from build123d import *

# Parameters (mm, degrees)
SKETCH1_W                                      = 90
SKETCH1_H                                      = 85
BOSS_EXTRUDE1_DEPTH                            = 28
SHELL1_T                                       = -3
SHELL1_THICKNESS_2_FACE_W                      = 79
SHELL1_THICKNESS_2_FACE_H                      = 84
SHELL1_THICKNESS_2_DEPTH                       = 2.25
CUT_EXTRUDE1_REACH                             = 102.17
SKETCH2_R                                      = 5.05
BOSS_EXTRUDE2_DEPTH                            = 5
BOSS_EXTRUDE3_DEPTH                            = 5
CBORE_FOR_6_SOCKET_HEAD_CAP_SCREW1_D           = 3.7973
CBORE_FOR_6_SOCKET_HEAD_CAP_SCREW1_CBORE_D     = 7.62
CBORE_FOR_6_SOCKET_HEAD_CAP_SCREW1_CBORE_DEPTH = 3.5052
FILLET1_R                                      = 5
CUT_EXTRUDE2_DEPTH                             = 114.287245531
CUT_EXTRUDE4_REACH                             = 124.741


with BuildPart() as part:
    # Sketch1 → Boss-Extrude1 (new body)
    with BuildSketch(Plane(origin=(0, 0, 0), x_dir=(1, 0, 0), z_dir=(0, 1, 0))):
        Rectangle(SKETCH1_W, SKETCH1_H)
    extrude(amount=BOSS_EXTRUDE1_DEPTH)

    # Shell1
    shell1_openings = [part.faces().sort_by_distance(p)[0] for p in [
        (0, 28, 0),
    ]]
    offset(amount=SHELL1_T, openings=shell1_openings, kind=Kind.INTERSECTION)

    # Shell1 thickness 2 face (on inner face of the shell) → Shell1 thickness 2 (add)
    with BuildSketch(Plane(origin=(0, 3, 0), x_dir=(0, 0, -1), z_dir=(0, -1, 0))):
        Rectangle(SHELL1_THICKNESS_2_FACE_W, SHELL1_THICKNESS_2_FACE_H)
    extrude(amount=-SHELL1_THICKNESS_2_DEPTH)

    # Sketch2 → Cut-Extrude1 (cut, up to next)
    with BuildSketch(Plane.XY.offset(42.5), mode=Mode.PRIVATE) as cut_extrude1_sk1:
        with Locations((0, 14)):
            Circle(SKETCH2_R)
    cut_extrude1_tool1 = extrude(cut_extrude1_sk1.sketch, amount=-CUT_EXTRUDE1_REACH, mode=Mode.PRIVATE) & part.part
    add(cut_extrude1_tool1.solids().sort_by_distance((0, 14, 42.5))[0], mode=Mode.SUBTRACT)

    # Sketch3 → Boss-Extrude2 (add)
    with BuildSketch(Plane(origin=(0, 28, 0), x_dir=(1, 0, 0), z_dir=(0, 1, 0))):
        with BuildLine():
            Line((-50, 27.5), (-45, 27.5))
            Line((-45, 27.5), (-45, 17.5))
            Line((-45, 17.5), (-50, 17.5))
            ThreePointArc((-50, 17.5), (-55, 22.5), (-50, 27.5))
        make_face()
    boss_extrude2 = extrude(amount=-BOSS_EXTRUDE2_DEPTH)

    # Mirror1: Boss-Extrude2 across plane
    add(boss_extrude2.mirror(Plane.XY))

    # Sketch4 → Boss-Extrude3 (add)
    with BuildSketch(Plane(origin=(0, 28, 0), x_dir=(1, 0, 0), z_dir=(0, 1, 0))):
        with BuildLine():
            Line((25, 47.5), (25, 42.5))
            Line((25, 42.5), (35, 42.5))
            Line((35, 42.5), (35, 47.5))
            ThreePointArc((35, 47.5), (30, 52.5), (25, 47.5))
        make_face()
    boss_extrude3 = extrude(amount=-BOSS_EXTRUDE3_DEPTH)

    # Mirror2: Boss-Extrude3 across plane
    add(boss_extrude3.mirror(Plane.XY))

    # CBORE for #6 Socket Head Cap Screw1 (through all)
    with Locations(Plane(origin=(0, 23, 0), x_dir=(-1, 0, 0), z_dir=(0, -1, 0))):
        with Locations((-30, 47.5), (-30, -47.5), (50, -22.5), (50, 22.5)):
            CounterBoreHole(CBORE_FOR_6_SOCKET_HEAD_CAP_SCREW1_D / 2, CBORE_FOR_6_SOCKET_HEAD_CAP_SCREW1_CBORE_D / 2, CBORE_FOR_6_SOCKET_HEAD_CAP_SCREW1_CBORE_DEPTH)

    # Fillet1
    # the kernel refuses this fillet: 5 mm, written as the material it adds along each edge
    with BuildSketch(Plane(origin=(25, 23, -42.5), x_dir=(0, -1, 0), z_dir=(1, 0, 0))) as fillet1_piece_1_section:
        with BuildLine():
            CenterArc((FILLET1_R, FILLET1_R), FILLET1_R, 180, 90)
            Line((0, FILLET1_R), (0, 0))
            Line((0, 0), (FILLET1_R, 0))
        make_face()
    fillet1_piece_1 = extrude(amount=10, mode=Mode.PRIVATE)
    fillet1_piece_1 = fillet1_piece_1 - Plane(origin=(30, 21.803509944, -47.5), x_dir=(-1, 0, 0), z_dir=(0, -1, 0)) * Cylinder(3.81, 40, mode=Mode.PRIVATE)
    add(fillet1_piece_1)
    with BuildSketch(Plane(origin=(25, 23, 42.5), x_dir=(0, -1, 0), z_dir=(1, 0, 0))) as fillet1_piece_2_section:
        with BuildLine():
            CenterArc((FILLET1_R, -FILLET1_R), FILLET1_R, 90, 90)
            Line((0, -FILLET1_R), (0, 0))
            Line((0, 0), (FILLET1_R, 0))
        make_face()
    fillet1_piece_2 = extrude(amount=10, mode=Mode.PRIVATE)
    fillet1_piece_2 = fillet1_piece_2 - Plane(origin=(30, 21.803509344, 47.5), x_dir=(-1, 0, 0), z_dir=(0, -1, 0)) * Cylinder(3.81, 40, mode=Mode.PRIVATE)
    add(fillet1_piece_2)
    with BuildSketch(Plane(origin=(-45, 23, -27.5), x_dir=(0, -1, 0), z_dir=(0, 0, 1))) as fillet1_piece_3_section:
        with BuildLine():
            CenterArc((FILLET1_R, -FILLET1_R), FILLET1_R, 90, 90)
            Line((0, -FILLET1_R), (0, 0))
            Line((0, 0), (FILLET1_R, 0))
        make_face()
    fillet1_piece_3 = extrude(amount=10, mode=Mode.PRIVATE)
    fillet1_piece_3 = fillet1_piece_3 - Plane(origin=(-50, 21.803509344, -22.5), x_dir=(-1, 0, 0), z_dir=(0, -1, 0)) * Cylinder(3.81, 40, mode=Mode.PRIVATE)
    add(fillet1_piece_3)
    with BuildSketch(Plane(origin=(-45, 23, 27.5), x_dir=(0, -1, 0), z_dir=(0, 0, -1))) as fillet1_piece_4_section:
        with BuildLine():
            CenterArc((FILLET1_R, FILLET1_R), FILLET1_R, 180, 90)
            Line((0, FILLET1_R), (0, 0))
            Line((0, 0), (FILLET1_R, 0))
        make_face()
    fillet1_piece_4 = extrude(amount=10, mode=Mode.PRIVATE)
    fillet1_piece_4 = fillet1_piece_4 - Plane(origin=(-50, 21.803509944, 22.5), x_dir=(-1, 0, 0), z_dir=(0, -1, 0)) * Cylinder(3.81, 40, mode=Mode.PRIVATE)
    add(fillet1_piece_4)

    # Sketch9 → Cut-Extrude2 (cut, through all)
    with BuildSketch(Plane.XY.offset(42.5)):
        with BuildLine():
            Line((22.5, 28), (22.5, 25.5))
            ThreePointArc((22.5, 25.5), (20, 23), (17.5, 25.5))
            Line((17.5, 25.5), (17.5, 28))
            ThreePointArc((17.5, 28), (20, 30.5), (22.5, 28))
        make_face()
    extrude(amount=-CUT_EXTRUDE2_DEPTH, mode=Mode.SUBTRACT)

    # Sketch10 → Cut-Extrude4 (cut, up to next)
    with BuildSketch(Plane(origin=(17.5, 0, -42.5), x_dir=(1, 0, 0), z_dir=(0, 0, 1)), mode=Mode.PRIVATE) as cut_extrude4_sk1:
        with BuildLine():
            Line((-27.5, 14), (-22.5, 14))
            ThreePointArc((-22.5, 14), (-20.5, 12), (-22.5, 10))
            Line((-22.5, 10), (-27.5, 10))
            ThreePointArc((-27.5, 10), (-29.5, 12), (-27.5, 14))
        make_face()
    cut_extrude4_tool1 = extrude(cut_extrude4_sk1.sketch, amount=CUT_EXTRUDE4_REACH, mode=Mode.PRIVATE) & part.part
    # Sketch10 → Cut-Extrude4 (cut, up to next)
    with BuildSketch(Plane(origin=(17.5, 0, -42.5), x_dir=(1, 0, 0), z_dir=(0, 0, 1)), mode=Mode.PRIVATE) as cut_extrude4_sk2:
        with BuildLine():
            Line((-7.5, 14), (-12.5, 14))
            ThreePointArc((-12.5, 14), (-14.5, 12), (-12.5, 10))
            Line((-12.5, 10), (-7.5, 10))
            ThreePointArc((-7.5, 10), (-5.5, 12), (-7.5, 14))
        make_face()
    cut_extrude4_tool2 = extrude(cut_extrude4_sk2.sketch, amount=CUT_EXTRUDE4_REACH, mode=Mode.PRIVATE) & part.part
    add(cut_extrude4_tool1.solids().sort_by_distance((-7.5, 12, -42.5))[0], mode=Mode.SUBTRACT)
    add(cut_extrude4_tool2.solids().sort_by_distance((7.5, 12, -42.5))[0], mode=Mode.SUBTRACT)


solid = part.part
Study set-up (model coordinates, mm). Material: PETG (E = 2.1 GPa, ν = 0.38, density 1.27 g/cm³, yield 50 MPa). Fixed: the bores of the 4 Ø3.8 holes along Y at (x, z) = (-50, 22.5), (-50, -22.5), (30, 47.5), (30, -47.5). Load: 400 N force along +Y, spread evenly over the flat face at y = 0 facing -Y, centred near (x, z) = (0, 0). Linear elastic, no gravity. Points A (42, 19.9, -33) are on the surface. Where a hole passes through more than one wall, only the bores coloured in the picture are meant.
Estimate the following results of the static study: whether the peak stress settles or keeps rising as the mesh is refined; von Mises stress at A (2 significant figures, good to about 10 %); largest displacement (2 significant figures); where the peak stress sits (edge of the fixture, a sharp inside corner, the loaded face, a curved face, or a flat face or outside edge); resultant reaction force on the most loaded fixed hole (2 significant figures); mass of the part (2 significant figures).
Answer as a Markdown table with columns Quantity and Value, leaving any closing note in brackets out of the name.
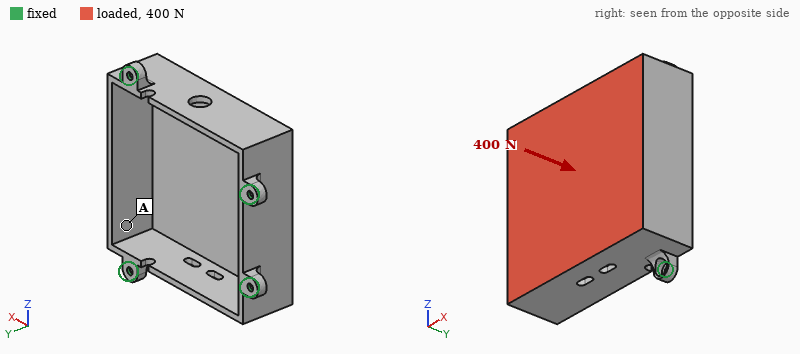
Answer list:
| Quantity | Value |
|---|---|
| whether the peak stress settles or keeps rising as the mesh is refined | keeps rising |
| von Mises stress at A | 1.7 MPa |
| largest displacement | 0.38 mm |
| where the peak stress sits | edge of the fixture |
| resultant reaction force on the most loaded fixed hole | 130 N |
| mass of the part | 81 g |
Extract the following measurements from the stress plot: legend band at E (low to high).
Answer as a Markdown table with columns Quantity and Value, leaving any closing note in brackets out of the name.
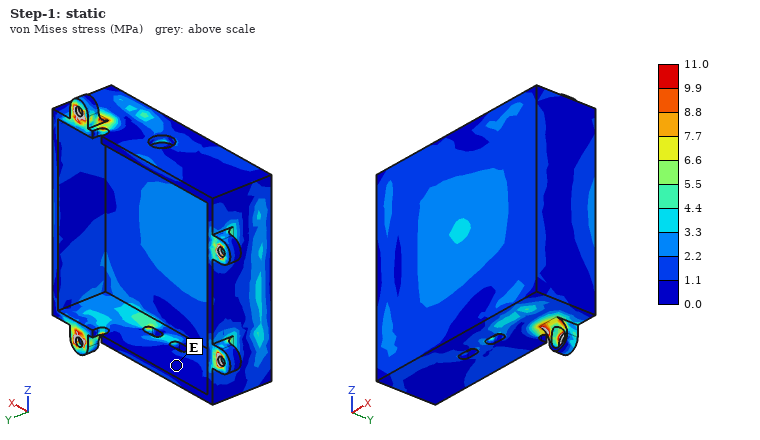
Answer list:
| Quantity | Value |
|---|---|
| legend band at E | 0.0 to 1.1 MPa |
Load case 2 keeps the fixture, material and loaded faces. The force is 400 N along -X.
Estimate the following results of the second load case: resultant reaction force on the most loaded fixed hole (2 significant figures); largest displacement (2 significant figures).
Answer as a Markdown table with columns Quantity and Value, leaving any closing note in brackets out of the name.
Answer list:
| Quantity | Value |
|---|---|
| resultant reaction force on the most loaded fixed hole | 160 N |
| largest displacement | 0.31 mm |
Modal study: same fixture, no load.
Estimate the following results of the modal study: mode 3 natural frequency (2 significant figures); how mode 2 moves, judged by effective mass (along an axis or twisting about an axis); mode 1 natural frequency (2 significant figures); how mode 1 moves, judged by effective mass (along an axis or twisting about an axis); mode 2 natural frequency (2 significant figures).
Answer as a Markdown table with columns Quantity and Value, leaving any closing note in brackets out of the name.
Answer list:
| Quantity | Value |
|---|---|
| mode 3 natural frequency | 870 Hz |
| how mode 2 moves, judged by effective mass | along X |
| mode 1 natural frequency | 670 Hz |
| how mode 1 moves, judged by effective mass | along Z |
| mode 2 natural frequency | 730 Hz |
